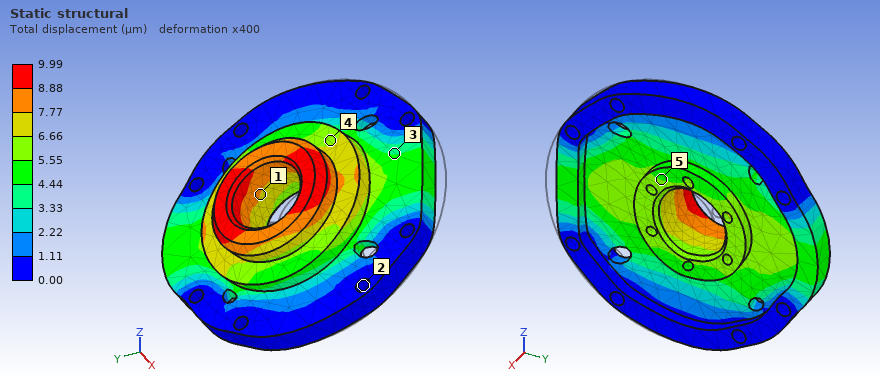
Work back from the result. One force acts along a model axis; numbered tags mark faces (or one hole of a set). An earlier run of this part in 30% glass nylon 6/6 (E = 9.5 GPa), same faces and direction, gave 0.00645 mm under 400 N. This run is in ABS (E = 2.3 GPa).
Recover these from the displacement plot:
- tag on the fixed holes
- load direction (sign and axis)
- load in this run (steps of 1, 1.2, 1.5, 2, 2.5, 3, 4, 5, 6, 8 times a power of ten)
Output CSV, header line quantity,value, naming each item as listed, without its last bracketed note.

quantity,value
tag on the fixed holes,2
load direction,+Y
load in this run,150 N
